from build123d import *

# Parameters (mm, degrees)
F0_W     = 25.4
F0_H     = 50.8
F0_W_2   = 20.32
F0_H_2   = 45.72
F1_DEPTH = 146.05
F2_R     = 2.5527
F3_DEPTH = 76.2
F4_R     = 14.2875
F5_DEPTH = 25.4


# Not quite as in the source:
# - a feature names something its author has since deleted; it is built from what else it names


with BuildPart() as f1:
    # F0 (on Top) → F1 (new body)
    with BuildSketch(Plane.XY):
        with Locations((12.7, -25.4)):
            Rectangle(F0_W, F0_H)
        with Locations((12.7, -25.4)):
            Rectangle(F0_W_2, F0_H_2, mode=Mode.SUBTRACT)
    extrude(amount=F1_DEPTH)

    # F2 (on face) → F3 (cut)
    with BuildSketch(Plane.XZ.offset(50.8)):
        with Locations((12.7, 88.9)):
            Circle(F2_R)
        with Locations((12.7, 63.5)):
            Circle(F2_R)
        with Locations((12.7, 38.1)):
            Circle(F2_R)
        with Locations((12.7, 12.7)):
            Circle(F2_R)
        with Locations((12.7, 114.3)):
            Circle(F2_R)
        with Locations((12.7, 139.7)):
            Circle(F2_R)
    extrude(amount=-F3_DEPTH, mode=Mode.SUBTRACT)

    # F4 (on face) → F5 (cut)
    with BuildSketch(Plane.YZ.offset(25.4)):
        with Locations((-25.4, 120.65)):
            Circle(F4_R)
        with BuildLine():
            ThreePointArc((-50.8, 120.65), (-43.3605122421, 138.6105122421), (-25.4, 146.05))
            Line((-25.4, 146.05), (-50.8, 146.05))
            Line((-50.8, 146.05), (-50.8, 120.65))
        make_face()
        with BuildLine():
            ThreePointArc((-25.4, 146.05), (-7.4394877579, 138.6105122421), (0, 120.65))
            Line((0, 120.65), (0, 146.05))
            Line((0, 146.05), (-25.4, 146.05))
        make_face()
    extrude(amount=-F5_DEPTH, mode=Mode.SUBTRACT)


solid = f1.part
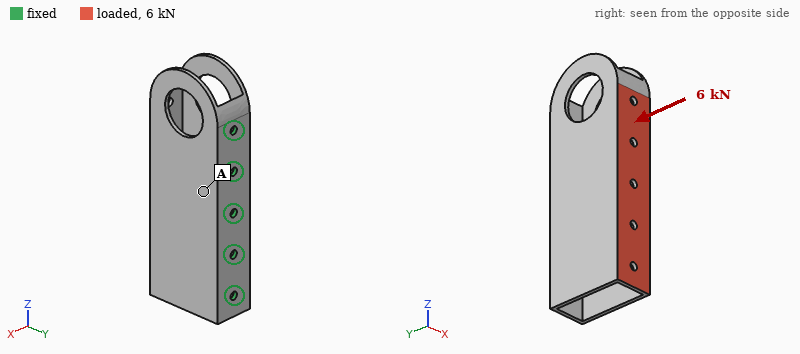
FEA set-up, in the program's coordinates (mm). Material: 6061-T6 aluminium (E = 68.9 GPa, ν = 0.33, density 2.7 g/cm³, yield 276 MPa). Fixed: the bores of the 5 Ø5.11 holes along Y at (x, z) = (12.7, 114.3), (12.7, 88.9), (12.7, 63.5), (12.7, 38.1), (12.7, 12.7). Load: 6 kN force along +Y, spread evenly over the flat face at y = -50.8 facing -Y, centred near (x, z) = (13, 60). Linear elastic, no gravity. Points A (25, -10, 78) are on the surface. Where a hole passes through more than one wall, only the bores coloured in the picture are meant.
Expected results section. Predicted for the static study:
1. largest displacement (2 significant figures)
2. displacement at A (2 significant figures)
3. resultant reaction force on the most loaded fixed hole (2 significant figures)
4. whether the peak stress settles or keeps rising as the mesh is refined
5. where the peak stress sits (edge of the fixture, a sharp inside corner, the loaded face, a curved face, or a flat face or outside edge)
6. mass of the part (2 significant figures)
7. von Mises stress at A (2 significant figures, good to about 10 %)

0.15 mm
0.099 mm
1.3 kN
keeps rising
edge of the fixture
120 g
25 MPa
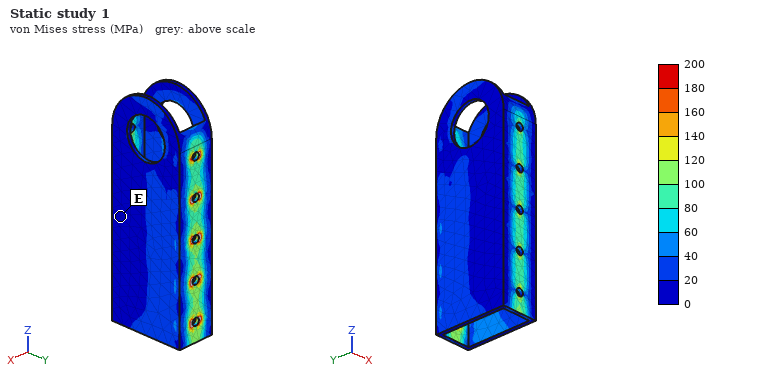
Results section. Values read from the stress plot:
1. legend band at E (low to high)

0 to 20 MPa
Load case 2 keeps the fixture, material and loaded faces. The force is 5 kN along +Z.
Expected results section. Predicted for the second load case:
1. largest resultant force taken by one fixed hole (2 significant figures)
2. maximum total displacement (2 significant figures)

2.2 kN
0.21 mm
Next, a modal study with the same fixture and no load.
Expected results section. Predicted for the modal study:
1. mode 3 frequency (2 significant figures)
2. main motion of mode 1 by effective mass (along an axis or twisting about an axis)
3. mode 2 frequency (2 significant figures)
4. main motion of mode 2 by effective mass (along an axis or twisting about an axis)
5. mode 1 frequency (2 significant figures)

2800 Hz
along X
2000 Hz
twisting about Y
700 Hz
